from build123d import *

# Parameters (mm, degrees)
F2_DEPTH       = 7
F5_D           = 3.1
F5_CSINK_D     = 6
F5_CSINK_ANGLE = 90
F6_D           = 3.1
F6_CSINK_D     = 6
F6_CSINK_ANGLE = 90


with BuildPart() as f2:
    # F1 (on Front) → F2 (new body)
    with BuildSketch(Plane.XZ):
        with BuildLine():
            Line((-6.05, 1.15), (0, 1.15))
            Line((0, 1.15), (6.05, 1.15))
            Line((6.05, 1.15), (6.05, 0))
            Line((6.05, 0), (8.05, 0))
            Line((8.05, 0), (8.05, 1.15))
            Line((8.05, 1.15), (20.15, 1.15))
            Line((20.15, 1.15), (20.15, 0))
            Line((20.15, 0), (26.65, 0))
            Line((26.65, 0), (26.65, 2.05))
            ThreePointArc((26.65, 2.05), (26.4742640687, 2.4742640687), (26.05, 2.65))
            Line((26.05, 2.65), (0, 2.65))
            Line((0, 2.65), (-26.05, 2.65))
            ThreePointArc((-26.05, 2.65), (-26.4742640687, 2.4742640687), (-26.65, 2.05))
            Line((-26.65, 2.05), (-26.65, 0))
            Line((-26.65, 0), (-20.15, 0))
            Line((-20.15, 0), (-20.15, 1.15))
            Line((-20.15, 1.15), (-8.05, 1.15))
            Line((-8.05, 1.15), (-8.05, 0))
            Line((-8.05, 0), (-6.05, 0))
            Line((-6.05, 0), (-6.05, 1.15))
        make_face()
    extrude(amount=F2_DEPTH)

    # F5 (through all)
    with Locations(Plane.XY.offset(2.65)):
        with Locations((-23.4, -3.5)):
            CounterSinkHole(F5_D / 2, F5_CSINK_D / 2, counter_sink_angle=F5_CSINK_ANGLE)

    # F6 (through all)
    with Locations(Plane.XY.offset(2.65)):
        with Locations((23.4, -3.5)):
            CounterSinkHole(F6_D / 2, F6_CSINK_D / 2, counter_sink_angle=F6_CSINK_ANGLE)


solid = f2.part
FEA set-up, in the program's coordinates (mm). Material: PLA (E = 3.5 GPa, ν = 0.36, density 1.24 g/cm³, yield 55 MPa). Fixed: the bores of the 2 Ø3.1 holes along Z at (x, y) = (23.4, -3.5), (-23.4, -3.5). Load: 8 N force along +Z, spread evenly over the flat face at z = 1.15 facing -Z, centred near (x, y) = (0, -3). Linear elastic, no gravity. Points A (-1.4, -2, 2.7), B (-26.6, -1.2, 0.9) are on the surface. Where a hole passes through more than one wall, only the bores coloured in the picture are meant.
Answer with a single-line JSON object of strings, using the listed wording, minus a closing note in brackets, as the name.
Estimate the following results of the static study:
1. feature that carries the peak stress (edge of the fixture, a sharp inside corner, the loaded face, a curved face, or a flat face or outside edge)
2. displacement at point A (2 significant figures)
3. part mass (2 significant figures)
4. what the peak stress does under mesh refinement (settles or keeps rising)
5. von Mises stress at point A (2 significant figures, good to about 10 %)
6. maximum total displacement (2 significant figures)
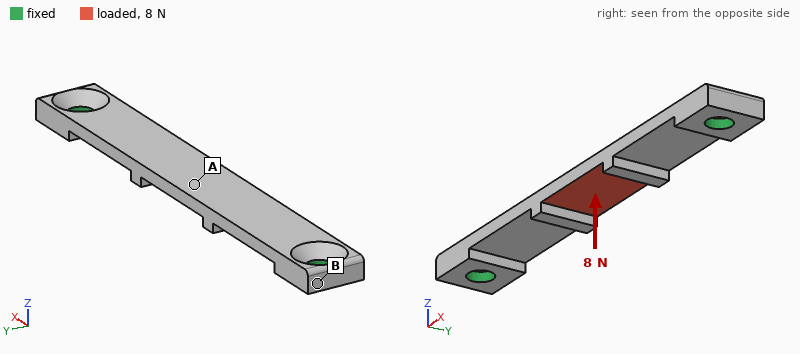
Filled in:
{"feature that carries the peak stress": "edge of the fixture", "displacement at point A": "0.44 mm", "part mass": "0.78 g", "what the peak stress does under mesh refinement": "keeps rising", "von Mises stress at point A": "13 MPa", "maximum total displacement": "0.45 mm"}
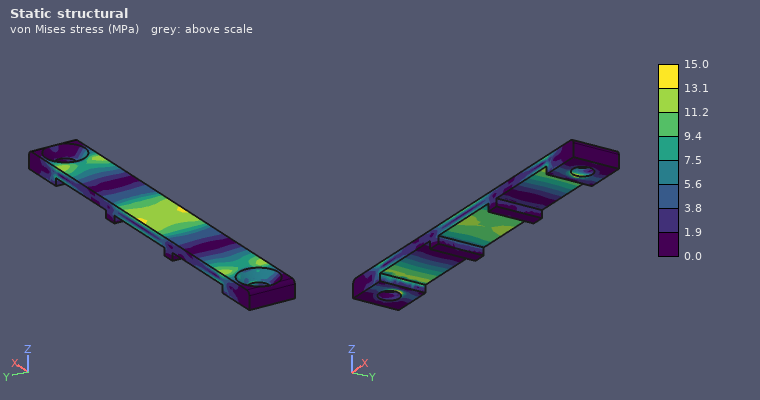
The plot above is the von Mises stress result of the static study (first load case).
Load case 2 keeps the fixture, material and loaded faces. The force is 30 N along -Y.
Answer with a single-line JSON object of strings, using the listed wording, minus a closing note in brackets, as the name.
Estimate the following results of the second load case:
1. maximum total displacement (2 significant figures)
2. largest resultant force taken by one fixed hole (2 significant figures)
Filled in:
{"maximum total displacement": "0.18 mm", "largest resultant force taken by one fixed hole": "15 N"}
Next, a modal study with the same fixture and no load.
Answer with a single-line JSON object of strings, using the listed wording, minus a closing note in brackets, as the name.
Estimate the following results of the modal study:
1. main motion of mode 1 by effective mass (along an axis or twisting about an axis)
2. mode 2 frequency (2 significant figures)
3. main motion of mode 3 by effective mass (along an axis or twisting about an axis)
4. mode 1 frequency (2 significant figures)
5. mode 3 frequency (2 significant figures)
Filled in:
{"main motion of mode 1 by effective mass": "along Z", "mode 2 frequency": "3600 Hz", "main motion of mode 3 by effective mass": "along Y", "mode 1 frequency": "1300 Hz", "mode 3 frequency": "4200 Hz"}
